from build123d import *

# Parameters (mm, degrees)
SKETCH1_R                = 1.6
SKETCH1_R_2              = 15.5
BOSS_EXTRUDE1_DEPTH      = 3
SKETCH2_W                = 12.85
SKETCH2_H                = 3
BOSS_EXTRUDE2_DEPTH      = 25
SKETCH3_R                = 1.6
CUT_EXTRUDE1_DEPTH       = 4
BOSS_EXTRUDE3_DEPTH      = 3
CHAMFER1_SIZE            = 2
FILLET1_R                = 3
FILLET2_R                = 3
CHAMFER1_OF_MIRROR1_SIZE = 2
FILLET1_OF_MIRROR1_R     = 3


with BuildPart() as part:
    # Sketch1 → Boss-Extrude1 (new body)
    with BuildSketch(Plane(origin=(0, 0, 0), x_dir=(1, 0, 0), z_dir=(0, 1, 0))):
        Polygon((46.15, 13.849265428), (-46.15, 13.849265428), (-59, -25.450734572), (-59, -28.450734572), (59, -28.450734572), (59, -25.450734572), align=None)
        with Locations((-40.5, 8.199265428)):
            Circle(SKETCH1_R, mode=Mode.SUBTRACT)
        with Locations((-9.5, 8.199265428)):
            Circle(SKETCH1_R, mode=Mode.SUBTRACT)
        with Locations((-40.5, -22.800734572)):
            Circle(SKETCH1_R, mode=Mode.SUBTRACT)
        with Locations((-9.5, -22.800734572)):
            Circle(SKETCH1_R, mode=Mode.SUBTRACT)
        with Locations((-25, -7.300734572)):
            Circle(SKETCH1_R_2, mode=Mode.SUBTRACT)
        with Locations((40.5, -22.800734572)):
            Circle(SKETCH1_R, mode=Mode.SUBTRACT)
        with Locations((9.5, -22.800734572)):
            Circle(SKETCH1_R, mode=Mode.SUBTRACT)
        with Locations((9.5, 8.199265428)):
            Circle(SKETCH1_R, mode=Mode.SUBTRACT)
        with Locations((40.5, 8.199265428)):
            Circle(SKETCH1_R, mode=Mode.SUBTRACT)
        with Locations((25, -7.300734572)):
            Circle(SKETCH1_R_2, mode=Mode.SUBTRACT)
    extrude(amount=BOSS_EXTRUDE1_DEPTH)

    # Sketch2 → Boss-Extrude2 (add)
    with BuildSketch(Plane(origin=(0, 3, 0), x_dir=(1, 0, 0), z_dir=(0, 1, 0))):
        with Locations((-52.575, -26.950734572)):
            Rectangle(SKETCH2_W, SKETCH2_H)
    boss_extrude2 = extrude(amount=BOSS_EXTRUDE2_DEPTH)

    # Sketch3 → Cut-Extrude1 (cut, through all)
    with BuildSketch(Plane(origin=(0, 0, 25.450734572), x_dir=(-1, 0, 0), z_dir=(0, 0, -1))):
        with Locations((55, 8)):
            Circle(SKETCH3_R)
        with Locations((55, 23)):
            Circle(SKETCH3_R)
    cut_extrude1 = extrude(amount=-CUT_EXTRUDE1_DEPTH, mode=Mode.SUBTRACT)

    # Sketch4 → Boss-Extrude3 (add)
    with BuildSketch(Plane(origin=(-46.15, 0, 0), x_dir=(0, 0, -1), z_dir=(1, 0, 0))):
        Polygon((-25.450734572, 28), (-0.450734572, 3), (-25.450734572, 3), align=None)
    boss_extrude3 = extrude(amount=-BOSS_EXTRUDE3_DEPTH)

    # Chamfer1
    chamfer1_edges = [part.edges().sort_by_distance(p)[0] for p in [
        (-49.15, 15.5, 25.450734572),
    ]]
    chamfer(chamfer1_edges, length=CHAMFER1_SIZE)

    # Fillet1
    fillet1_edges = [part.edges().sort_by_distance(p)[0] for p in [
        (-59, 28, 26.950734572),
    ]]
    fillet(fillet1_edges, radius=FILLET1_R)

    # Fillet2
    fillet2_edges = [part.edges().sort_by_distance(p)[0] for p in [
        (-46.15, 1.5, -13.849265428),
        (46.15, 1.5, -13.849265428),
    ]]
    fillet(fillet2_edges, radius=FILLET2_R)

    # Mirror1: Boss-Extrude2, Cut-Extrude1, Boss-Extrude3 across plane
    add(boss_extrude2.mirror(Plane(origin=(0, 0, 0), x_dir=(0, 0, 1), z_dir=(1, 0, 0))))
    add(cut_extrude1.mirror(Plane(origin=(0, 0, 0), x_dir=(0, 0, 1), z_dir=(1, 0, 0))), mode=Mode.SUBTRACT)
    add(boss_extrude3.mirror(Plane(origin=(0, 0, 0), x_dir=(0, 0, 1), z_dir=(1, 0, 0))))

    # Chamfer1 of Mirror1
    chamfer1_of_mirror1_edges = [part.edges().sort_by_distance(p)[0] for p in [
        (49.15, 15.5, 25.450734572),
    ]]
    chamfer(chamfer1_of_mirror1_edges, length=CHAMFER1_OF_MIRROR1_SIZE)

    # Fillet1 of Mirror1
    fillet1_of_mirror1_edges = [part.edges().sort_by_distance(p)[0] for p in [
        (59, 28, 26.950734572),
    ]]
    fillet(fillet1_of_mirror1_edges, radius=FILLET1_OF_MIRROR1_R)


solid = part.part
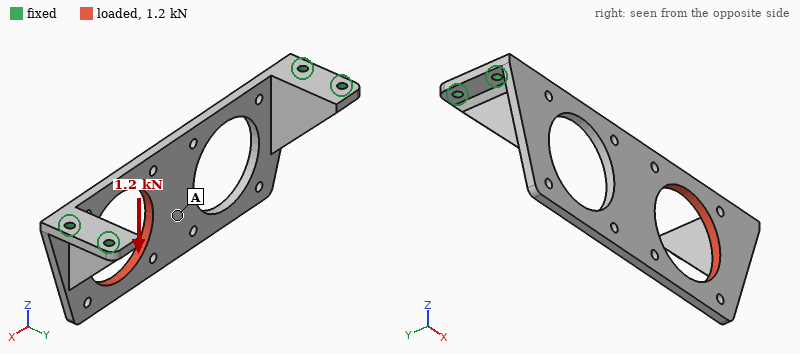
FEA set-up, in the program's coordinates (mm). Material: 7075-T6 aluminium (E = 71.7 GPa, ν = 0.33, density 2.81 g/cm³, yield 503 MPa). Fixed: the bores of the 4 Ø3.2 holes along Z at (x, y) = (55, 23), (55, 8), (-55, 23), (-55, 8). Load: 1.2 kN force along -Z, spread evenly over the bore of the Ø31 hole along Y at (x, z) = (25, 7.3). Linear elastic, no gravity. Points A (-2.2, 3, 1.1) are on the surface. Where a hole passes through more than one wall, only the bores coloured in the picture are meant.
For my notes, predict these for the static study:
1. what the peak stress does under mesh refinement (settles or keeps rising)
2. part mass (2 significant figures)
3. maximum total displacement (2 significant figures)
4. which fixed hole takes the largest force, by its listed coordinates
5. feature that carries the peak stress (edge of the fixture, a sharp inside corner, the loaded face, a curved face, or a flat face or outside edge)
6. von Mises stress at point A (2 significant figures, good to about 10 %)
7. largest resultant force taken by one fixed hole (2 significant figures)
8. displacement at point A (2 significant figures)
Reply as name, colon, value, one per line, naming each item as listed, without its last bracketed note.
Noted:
what the peak stress does under mesh refinement: keeps rising
part mass: 35 g
maximum total displacement: 98 µm
which fixed hole takes the largest force, by its listed coordinates: (55, 8)
feature that carries the peak stress: edge of the fixture
von Mises stress at point A: 10 MPa
largest resultant force taken by one fixed hole: 1.2 kN
displacement at point A: 81 µm
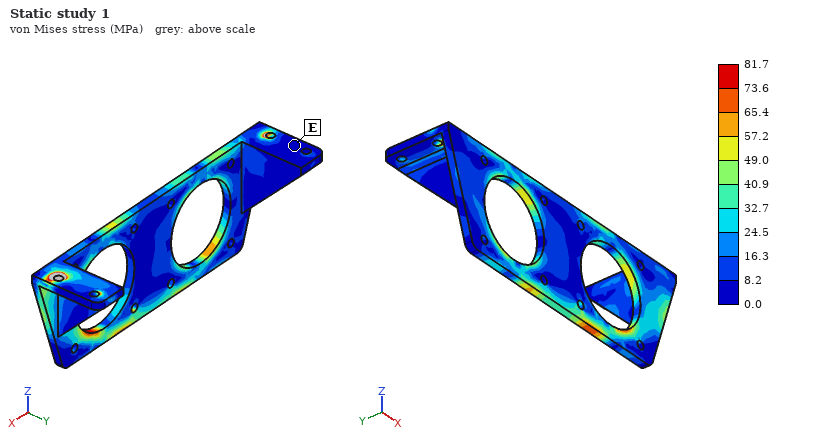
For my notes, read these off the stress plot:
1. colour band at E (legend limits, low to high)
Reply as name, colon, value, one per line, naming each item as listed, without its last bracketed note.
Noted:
colour band at E: 0.0 to 8.2 MPa
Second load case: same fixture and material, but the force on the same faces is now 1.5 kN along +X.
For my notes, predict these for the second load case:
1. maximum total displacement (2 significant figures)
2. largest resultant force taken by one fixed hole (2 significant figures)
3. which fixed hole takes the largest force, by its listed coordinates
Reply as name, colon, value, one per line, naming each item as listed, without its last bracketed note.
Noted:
maximum total displacement: 55 µm
largest resultant force taken by one fixed hole: 1.2 kN
which fixed hole takes the largest force, by its listed coordinates: (55, 8)
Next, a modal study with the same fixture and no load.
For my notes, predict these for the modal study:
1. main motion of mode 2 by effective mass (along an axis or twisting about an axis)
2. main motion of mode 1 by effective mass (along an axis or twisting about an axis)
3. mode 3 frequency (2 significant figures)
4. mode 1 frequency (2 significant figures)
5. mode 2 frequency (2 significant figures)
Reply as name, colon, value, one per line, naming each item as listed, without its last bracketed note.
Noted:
main motion of mode 2 by effective mass: twisting about X
main motion of mode 1 by effective mass: along Y
mode 3 frequency: 3400 Hz
mode 1 frequency: 1200 Hz
mode 2 frequency: 2000 Hz
